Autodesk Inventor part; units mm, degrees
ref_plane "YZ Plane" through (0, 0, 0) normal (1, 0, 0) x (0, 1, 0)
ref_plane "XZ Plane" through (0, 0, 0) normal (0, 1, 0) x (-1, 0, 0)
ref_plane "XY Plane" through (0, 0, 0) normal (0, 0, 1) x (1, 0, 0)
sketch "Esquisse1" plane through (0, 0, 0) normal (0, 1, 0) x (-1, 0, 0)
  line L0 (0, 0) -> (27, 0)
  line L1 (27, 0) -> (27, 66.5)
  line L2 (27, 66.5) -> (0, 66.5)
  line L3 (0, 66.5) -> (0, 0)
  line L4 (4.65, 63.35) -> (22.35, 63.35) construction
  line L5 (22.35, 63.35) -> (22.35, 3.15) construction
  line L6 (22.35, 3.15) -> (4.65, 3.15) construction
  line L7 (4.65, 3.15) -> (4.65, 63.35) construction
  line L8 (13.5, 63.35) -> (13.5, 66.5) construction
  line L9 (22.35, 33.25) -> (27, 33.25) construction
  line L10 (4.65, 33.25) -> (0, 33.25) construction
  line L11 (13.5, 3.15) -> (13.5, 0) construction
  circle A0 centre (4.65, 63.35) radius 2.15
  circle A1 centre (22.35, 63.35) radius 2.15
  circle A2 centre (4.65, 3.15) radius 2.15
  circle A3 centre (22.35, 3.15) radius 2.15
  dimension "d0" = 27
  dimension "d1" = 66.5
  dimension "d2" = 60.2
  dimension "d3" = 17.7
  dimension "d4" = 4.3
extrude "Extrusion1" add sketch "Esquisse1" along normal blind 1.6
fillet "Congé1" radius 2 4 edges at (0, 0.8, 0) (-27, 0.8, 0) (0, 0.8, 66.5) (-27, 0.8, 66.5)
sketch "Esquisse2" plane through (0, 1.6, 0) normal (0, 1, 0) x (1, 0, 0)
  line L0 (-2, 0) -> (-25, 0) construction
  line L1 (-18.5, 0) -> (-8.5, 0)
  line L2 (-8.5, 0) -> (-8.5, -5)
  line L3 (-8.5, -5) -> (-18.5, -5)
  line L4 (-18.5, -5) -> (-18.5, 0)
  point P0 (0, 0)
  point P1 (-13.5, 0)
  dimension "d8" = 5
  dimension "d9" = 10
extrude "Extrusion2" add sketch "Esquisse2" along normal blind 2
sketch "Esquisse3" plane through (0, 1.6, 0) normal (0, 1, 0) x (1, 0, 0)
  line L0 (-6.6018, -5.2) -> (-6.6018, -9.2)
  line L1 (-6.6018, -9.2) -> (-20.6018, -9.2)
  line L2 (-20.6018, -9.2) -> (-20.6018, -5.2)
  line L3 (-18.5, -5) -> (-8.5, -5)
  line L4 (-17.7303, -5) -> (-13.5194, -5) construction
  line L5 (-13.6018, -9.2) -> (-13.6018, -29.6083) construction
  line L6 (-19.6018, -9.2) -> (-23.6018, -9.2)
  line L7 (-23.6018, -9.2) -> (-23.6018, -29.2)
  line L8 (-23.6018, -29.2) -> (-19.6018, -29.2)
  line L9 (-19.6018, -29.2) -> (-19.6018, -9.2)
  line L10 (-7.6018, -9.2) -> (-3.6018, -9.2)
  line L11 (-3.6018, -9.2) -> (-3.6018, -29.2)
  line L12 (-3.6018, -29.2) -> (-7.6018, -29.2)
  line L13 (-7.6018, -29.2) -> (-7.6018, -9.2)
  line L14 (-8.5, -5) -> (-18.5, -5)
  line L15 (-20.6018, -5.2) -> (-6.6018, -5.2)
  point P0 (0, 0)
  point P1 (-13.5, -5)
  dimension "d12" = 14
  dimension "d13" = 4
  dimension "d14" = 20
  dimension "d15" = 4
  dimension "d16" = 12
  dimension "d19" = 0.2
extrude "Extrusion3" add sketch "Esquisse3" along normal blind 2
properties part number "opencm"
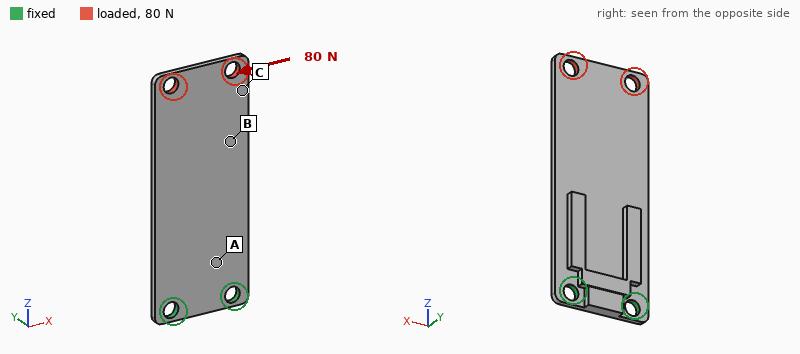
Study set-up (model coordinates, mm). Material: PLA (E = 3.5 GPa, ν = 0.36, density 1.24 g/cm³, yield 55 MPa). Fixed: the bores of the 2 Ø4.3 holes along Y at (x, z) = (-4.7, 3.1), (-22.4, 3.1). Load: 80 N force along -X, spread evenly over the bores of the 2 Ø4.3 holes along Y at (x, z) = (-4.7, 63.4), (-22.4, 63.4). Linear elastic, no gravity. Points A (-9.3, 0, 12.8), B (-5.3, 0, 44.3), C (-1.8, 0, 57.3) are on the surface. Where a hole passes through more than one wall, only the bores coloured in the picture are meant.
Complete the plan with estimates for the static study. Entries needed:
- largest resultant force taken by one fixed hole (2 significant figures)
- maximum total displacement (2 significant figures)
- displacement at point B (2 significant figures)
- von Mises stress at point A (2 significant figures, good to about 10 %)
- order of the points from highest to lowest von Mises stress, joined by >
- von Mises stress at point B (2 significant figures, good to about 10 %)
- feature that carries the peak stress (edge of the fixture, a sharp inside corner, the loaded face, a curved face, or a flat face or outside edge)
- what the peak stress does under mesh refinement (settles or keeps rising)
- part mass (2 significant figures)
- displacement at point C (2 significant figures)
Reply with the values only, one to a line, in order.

250 N
0.75 mm
0.38 mm
9.3 MPa
A > B > C
5.3 MPa
edge of the fixture
keeps rising
4.1 g
0.59 mm
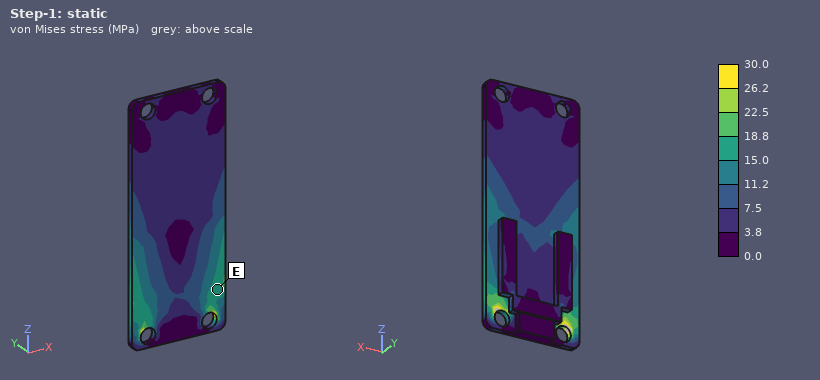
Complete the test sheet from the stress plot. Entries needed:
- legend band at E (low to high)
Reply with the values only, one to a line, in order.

15.0 to 18.8 MPa
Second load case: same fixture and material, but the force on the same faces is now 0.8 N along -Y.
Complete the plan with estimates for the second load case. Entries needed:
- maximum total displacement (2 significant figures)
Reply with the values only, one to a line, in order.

0.85 mm
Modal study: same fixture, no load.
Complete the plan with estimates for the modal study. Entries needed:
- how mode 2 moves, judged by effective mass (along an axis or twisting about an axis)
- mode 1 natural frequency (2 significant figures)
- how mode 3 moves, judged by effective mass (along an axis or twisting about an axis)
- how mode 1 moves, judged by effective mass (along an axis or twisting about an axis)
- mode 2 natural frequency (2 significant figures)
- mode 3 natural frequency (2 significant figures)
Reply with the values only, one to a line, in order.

twisting about Z
180 Hz
along Y
along Y
710 Hz
790 Hz
